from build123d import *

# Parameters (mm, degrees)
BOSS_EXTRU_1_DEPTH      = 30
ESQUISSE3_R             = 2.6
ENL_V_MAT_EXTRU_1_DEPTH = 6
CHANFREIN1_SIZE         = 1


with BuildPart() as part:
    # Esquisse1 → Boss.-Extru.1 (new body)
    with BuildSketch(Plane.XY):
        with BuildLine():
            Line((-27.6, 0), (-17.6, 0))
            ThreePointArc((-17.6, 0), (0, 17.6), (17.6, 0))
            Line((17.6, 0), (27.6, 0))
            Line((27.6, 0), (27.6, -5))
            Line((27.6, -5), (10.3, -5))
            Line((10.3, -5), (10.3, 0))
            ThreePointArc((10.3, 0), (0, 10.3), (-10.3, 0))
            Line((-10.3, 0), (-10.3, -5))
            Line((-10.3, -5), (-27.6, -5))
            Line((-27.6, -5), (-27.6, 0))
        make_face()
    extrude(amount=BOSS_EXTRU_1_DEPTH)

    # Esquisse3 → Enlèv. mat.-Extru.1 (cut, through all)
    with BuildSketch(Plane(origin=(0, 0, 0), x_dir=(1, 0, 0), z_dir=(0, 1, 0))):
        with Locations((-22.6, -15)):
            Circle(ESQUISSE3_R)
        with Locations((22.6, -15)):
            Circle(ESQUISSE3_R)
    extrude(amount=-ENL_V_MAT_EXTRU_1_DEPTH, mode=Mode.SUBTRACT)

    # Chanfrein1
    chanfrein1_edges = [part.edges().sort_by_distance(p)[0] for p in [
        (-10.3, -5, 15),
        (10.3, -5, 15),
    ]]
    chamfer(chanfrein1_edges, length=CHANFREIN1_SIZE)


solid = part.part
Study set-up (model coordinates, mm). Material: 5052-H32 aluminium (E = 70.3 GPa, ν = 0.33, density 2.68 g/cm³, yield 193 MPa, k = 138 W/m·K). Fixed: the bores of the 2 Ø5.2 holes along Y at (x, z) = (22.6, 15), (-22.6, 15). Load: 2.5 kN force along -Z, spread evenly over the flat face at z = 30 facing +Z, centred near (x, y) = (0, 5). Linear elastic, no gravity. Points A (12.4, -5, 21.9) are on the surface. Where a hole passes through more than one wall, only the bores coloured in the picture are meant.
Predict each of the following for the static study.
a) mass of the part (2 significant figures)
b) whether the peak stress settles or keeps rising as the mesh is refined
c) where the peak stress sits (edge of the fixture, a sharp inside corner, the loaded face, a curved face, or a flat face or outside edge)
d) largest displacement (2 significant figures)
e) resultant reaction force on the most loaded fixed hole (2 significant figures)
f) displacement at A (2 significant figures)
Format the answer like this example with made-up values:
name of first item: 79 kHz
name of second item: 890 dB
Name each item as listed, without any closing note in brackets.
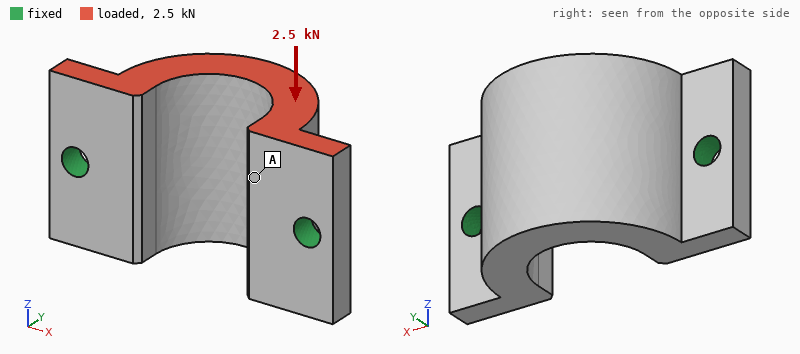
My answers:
mass of the part: 39 g
whether the peak stress settles or keeps rising as the mesh is refined: keeps rising
where the peak stress sits: edge of the fixture
largest displacement: 69 µm
resultant reaction force on the most loaded fixed hole: 1.3 kN
displacement at A: 17 µm
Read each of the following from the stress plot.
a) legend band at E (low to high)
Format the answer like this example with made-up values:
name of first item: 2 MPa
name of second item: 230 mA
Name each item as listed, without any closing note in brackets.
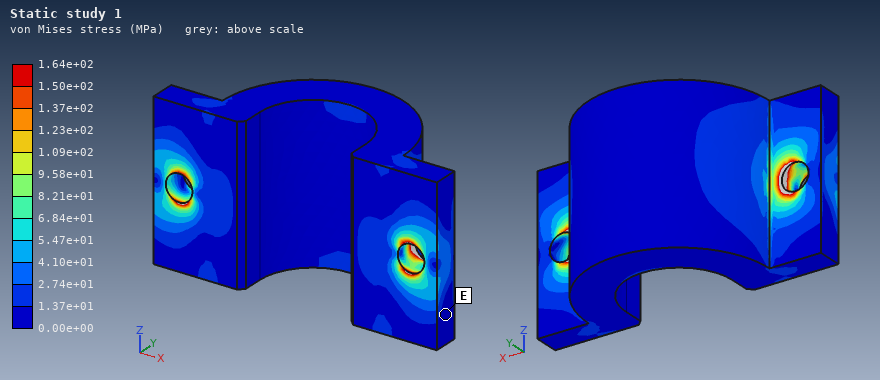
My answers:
legend band at E: 0.00e+00 to 1.37e+01 MPa
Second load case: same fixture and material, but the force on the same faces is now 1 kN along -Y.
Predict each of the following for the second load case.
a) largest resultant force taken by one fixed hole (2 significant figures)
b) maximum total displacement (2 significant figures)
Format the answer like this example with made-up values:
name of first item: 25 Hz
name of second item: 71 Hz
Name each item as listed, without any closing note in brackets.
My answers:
largest resultant force taken by one fixed hole: 550 N
maximum total displacement: 45 µm
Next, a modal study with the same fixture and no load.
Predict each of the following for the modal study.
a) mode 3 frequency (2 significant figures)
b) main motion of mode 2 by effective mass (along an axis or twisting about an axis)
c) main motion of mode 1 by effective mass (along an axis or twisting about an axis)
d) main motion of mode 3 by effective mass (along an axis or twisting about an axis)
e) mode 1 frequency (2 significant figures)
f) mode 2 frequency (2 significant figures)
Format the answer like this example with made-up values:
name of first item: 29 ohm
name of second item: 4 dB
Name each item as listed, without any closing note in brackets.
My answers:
mode 3 frequency: 16 kHz
main motion of mode 2 by effective mass: along Y
main motion of mode 1 by effective mass: along Z
main motion of mode 3 by effective mass: along X
mode 1 frequency: 5400 Hz
mode 2 frequency: 15 kHz
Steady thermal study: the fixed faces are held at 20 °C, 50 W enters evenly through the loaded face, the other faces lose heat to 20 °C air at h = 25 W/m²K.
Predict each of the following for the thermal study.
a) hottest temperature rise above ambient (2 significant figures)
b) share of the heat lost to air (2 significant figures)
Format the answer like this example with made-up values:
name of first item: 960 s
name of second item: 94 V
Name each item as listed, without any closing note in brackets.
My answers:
hottest temperature rise above ambient: 25 K
share of the heat lost to air: 3.2 %
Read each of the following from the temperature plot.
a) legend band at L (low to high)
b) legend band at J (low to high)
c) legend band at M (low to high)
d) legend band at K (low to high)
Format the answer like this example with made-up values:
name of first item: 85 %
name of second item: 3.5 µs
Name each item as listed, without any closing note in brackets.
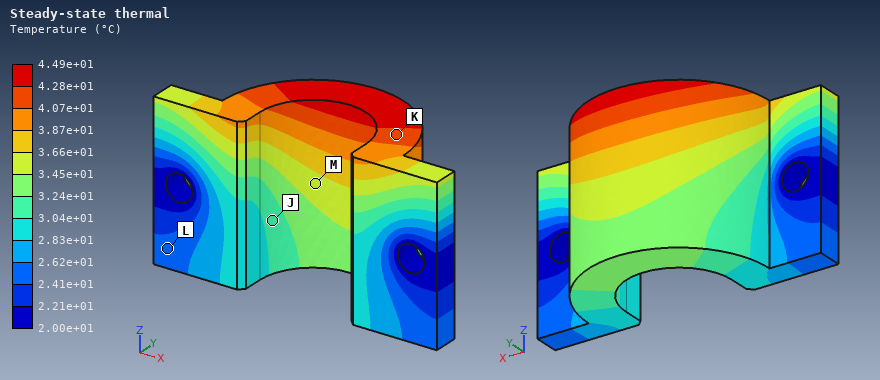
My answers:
legend band at L: 2.41e+01 to 2.62e+01 °C
legend band at J: 3.04e+01 to 3.24e+01 °C
legend band at M: 3.45e+01 to 3.66e+01 °C
legend band at K: 4.07e+01 to 4.28e+01 °C
